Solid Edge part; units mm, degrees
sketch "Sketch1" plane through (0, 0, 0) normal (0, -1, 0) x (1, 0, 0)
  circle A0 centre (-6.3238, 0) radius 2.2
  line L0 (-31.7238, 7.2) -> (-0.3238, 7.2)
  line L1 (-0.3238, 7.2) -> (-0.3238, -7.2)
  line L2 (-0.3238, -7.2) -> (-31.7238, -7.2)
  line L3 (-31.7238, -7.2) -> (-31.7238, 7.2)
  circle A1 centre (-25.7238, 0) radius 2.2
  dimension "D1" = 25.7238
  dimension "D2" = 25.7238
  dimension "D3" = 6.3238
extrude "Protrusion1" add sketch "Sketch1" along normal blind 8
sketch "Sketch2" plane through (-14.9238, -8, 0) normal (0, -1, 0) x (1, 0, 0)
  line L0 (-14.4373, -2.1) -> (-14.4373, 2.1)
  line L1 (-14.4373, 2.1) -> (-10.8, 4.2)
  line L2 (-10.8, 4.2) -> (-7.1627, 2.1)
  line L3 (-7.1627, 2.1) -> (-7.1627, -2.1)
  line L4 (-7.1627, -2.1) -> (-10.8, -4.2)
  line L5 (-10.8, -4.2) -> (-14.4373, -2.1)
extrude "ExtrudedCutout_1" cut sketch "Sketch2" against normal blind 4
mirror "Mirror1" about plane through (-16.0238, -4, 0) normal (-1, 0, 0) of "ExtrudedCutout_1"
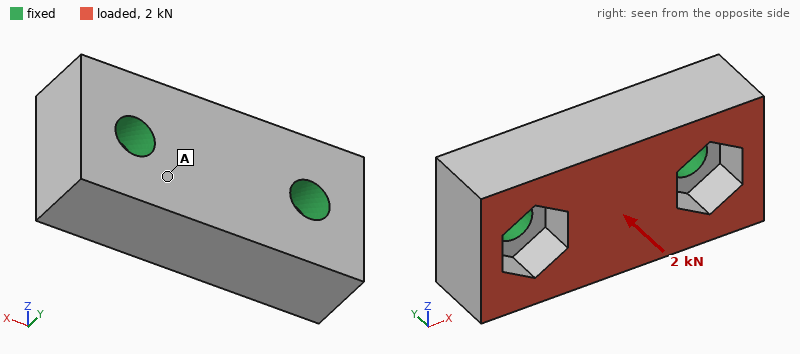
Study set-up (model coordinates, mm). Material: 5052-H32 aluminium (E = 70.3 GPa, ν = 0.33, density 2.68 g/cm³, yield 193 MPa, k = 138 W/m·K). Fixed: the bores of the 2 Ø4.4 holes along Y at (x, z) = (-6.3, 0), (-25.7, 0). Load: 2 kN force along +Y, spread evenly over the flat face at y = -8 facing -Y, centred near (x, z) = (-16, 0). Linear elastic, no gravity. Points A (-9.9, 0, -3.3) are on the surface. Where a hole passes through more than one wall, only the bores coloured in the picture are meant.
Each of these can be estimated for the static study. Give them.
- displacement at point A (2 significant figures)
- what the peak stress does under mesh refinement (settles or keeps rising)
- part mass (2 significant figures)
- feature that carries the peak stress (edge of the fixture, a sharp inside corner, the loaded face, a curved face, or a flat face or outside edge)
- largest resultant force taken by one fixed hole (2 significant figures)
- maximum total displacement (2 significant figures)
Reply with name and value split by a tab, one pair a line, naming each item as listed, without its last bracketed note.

displacement at point A	2.1 µm
what the peak stress does under mesh refinement	keeps rising
part mass	8.4 g
feature that carries the peak stress	edge of the fixture
largest resultant force taken by one fixed hole	1.0 kN
maximum total displacement	3.8 µm
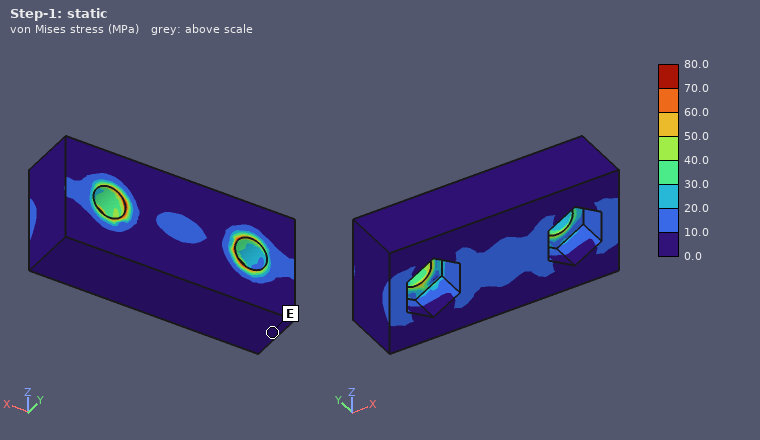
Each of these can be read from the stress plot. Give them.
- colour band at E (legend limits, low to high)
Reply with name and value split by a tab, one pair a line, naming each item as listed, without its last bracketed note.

colour band at E	0.0 to 10.0 MPa
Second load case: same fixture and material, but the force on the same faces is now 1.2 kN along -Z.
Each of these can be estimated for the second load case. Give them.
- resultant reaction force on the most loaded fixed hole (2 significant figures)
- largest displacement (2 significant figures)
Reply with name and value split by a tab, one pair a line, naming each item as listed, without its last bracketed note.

resultant reaction force on the most loaded fixed hole	600 N
largest displacement	10 µm
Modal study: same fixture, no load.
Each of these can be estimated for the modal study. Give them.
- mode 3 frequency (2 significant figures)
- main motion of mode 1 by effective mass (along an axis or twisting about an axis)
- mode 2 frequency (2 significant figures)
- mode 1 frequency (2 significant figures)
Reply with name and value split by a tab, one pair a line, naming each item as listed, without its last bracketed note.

mode 3 frequency	48 kHz
main motion of mode 1 by effective mass	along Z
mode 2 frequency	47 kHz
mode 1 frequency	32 kHz
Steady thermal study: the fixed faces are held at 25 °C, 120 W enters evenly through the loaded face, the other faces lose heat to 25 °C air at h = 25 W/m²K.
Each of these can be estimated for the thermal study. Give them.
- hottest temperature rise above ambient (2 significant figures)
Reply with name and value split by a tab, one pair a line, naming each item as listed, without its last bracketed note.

hottest temperature rise above ambient	33 K
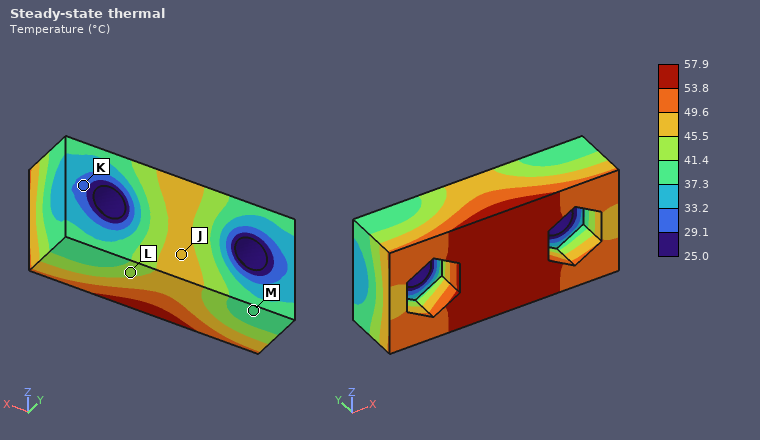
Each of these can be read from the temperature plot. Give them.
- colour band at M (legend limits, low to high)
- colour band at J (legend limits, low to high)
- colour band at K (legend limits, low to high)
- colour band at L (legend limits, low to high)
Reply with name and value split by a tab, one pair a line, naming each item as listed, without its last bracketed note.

colour band at M	37.3 to 41.4 °C
colour band at J	45.5 to 49.6 °C
colour band at K	29.1 to 33.2 °C
colour band at L	41.4 to 45.5 °C
